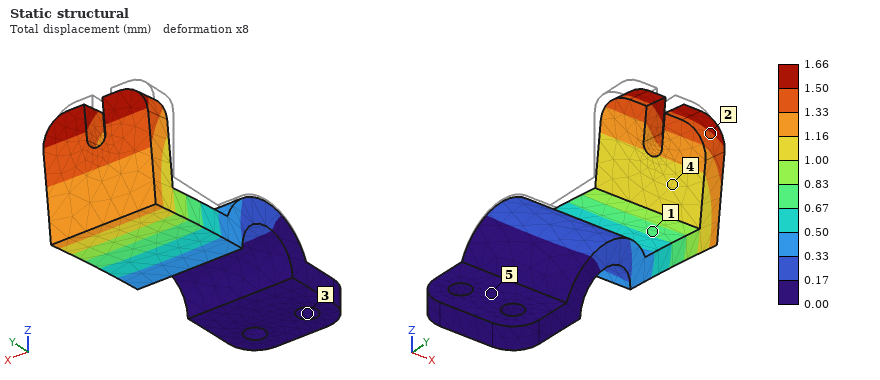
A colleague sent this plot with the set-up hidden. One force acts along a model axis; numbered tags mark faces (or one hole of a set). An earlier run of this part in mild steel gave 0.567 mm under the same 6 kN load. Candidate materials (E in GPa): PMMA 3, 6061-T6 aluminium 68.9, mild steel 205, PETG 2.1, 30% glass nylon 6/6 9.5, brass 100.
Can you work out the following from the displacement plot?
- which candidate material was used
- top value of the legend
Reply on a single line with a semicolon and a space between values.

6061-T6 aluminium; 1.66 mm
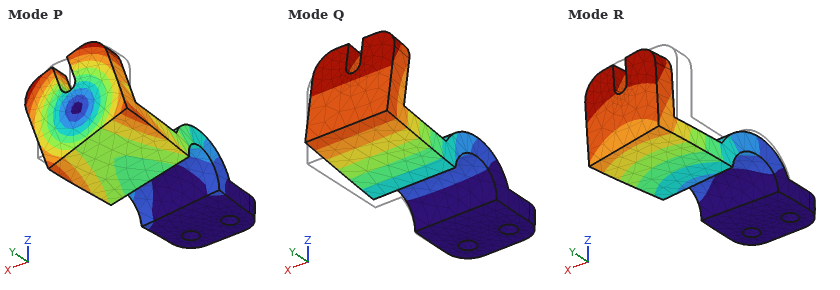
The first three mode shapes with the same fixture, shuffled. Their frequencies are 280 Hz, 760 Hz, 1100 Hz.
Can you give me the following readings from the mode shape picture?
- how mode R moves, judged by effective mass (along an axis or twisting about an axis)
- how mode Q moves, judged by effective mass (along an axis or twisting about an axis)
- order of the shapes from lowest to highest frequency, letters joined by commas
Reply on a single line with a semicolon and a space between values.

along X; along Z; Q, R, P
